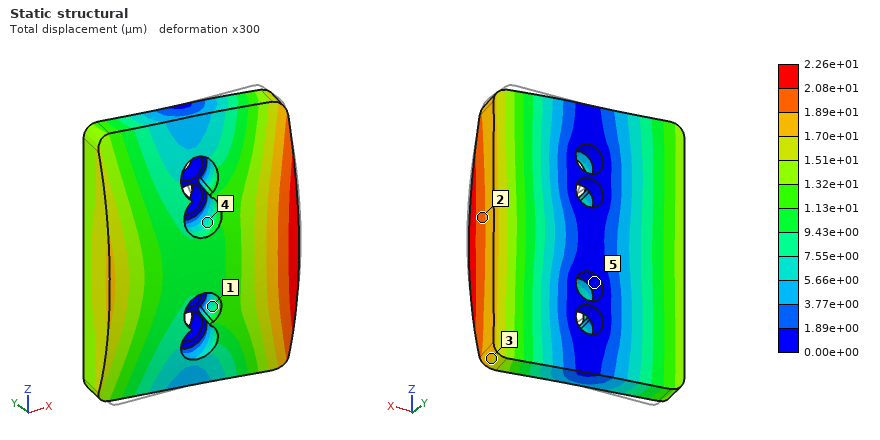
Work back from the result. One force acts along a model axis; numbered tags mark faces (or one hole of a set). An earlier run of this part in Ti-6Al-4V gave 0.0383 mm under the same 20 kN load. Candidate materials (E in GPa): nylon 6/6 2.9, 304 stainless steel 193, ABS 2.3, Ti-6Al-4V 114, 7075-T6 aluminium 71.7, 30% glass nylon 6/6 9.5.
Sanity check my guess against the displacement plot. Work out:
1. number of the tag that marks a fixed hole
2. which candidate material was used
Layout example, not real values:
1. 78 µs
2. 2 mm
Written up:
1. 5
2. 304 stainless steel
